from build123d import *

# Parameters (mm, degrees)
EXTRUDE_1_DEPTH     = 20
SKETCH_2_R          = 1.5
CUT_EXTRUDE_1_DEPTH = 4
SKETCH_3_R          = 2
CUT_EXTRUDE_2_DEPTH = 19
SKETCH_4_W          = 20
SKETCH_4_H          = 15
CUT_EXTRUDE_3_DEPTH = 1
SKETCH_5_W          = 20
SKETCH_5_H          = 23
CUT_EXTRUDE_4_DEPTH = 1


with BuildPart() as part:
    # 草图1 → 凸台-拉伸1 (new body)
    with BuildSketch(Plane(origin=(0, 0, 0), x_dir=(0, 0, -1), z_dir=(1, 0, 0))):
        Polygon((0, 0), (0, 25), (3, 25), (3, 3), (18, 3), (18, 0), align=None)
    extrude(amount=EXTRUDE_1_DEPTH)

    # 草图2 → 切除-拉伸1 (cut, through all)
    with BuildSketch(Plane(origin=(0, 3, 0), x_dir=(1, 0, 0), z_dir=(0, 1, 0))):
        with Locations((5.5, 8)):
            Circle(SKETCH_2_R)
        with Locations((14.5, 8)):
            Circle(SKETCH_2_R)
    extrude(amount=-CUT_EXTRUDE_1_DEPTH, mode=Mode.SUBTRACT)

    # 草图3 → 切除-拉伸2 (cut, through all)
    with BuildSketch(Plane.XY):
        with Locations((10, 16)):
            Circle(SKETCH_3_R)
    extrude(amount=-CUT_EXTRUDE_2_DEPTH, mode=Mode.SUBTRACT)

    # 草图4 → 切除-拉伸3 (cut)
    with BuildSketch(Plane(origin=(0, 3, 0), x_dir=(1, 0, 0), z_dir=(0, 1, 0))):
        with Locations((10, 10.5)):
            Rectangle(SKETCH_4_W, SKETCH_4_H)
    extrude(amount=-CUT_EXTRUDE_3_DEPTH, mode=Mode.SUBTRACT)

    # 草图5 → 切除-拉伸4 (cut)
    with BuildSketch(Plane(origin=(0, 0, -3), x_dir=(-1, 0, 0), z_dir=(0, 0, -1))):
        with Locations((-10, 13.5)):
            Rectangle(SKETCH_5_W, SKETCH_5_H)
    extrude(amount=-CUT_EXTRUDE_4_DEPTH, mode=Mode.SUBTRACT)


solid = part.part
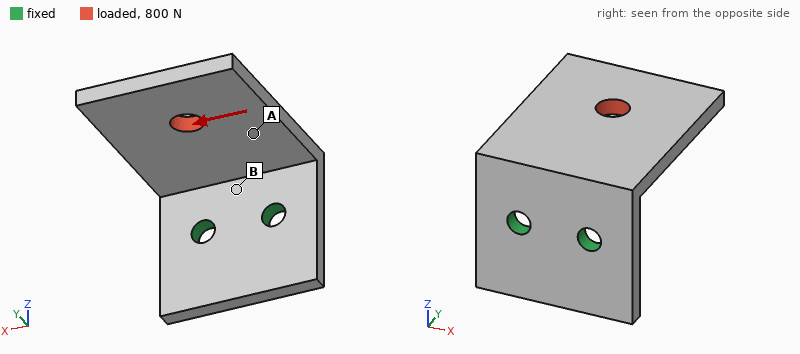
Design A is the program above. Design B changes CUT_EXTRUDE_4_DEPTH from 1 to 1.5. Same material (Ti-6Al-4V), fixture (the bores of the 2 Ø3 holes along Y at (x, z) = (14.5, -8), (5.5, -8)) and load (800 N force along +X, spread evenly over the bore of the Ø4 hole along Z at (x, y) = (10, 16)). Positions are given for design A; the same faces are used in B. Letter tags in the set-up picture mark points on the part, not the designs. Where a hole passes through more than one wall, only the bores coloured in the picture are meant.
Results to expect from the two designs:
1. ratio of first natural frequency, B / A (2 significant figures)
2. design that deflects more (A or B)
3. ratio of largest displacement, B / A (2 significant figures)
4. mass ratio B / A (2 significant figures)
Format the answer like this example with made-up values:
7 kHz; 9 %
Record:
0.90; B; 1.3; 0.86
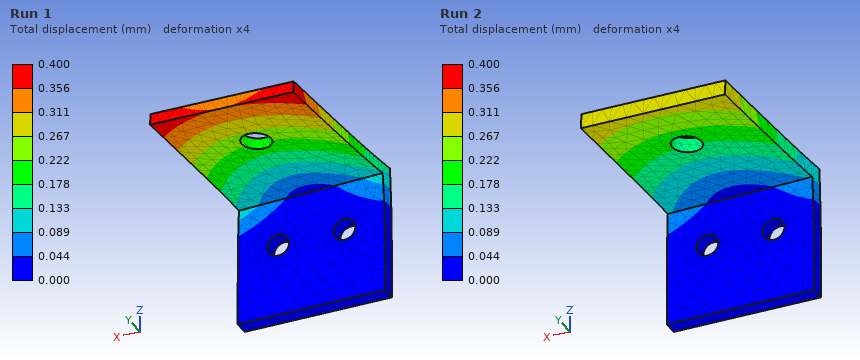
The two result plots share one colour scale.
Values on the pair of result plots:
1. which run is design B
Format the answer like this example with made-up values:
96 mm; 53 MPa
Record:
Run 1
